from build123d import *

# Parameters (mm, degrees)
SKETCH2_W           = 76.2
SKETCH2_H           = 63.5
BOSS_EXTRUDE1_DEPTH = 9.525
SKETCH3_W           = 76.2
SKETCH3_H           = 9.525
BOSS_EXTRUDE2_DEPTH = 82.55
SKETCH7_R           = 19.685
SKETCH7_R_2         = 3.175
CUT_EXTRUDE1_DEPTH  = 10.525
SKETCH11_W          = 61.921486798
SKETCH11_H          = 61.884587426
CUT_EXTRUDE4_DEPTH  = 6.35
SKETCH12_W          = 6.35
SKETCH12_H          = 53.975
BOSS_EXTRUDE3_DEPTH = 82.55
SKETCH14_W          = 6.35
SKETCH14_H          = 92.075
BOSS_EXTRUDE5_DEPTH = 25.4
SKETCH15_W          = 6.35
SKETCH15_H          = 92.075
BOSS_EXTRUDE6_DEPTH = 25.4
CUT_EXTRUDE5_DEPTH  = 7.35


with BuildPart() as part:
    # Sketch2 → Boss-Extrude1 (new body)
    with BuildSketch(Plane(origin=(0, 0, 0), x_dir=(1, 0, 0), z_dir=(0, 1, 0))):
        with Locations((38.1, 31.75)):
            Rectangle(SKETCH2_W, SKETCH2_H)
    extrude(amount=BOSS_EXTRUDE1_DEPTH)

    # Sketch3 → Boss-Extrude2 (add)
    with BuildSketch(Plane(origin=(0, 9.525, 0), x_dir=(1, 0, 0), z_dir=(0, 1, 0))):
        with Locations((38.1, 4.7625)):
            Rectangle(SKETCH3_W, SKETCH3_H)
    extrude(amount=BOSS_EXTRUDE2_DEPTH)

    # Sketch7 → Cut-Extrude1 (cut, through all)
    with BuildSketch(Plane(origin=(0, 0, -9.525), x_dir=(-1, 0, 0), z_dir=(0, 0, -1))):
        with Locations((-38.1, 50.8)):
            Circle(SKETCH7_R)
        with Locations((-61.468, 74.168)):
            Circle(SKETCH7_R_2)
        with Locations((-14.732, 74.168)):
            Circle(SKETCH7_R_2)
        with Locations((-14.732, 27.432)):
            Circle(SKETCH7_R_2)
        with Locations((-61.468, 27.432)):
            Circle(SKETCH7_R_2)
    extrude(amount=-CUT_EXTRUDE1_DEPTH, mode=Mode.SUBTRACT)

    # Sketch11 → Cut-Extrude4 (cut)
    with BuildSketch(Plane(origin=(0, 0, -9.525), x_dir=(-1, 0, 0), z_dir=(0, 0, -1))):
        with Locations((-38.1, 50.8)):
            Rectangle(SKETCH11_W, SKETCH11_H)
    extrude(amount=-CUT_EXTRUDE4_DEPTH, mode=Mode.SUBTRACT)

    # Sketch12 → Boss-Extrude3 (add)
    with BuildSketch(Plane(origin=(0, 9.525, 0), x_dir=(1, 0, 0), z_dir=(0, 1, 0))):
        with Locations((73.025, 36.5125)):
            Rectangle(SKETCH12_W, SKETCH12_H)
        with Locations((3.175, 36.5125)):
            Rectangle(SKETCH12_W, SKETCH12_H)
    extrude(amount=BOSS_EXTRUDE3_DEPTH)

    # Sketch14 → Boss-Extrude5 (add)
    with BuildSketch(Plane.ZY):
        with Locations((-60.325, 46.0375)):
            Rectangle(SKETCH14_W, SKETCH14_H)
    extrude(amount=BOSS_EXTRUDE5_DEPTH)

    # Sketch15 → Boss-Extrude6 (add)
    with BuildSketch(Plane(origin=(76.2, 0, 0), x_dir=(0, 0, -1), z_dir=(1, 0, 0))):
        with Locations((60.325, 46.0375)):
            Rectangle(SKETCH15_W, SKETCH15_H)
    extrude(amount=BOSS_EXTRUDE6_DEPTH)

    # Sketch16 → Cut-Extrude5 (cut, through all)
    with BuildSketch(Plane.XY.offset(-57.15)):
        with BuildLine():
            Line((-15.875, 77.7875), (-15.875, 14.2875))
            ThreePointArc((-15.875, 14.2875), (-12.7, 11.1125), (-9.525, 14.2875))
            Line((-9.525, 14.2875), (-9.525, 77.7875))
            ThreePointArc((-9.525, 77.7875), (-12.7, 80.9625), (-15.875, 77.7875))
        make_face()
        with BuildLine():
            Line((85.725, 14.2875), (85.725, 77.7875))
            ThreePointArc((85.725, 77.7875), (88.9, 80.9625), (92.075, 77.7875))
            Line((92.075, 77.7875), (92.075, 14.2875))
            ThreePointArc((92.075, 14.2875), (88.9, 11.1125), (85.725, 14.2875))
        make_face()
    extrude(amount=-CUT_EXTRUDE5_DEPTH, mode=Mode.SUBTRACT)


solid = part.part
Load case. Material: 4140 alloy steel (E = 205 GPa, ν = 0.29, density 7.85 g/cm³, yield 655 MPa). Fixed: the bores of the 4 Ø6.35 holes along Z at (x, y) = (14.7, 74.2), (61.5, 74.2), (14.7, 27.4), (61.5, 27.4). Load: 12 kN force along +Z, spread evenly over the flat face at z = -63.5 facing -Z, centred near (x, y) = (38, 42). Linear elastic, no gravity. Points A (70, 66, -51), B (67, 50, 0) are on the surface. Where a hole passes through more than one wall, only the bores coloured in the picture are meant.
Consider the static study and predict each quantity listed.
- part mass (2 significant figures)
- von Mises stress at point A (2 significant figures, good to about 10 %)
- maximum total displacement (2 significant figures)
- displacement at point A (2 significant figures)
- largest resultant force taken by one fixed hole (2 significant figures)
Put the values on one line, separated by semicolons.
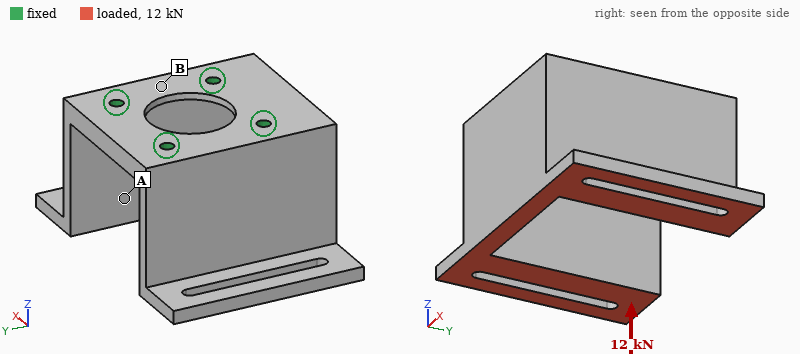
1.2 kg; 66 MPa; 0.31 mm; 0.093 mm; 4.1 kN
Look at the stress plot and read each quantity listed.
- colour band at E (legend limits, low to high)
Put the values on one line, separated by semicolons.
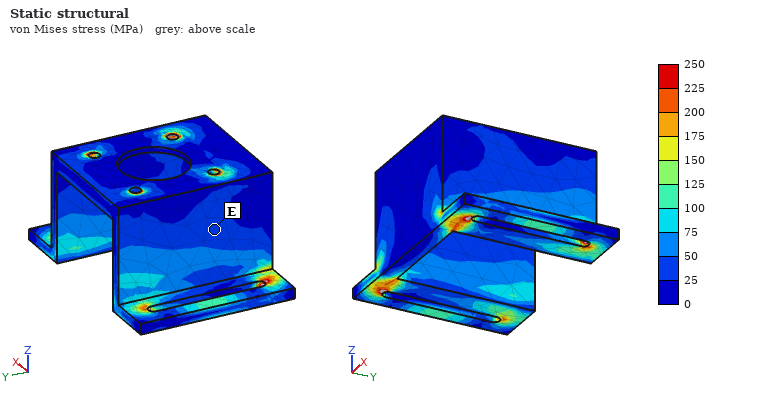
25 to 50 MPa
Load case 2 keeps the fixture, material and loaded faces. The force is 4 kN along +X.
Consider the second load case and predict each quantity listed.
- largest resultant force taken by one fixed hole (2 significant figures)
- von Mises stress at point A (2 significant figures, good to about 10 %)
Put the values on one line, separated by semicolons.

5.5 kN; 41 MPa
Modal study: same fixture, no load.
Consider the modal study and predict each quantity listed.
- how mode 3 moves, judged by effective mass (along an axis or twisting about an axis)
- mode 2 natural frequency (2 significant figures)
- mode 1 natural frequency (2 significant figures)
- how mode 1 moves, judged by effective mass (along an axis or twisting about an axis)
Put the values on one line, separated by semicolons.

along Y; 1200 Hz; 1100 Hz; along X
